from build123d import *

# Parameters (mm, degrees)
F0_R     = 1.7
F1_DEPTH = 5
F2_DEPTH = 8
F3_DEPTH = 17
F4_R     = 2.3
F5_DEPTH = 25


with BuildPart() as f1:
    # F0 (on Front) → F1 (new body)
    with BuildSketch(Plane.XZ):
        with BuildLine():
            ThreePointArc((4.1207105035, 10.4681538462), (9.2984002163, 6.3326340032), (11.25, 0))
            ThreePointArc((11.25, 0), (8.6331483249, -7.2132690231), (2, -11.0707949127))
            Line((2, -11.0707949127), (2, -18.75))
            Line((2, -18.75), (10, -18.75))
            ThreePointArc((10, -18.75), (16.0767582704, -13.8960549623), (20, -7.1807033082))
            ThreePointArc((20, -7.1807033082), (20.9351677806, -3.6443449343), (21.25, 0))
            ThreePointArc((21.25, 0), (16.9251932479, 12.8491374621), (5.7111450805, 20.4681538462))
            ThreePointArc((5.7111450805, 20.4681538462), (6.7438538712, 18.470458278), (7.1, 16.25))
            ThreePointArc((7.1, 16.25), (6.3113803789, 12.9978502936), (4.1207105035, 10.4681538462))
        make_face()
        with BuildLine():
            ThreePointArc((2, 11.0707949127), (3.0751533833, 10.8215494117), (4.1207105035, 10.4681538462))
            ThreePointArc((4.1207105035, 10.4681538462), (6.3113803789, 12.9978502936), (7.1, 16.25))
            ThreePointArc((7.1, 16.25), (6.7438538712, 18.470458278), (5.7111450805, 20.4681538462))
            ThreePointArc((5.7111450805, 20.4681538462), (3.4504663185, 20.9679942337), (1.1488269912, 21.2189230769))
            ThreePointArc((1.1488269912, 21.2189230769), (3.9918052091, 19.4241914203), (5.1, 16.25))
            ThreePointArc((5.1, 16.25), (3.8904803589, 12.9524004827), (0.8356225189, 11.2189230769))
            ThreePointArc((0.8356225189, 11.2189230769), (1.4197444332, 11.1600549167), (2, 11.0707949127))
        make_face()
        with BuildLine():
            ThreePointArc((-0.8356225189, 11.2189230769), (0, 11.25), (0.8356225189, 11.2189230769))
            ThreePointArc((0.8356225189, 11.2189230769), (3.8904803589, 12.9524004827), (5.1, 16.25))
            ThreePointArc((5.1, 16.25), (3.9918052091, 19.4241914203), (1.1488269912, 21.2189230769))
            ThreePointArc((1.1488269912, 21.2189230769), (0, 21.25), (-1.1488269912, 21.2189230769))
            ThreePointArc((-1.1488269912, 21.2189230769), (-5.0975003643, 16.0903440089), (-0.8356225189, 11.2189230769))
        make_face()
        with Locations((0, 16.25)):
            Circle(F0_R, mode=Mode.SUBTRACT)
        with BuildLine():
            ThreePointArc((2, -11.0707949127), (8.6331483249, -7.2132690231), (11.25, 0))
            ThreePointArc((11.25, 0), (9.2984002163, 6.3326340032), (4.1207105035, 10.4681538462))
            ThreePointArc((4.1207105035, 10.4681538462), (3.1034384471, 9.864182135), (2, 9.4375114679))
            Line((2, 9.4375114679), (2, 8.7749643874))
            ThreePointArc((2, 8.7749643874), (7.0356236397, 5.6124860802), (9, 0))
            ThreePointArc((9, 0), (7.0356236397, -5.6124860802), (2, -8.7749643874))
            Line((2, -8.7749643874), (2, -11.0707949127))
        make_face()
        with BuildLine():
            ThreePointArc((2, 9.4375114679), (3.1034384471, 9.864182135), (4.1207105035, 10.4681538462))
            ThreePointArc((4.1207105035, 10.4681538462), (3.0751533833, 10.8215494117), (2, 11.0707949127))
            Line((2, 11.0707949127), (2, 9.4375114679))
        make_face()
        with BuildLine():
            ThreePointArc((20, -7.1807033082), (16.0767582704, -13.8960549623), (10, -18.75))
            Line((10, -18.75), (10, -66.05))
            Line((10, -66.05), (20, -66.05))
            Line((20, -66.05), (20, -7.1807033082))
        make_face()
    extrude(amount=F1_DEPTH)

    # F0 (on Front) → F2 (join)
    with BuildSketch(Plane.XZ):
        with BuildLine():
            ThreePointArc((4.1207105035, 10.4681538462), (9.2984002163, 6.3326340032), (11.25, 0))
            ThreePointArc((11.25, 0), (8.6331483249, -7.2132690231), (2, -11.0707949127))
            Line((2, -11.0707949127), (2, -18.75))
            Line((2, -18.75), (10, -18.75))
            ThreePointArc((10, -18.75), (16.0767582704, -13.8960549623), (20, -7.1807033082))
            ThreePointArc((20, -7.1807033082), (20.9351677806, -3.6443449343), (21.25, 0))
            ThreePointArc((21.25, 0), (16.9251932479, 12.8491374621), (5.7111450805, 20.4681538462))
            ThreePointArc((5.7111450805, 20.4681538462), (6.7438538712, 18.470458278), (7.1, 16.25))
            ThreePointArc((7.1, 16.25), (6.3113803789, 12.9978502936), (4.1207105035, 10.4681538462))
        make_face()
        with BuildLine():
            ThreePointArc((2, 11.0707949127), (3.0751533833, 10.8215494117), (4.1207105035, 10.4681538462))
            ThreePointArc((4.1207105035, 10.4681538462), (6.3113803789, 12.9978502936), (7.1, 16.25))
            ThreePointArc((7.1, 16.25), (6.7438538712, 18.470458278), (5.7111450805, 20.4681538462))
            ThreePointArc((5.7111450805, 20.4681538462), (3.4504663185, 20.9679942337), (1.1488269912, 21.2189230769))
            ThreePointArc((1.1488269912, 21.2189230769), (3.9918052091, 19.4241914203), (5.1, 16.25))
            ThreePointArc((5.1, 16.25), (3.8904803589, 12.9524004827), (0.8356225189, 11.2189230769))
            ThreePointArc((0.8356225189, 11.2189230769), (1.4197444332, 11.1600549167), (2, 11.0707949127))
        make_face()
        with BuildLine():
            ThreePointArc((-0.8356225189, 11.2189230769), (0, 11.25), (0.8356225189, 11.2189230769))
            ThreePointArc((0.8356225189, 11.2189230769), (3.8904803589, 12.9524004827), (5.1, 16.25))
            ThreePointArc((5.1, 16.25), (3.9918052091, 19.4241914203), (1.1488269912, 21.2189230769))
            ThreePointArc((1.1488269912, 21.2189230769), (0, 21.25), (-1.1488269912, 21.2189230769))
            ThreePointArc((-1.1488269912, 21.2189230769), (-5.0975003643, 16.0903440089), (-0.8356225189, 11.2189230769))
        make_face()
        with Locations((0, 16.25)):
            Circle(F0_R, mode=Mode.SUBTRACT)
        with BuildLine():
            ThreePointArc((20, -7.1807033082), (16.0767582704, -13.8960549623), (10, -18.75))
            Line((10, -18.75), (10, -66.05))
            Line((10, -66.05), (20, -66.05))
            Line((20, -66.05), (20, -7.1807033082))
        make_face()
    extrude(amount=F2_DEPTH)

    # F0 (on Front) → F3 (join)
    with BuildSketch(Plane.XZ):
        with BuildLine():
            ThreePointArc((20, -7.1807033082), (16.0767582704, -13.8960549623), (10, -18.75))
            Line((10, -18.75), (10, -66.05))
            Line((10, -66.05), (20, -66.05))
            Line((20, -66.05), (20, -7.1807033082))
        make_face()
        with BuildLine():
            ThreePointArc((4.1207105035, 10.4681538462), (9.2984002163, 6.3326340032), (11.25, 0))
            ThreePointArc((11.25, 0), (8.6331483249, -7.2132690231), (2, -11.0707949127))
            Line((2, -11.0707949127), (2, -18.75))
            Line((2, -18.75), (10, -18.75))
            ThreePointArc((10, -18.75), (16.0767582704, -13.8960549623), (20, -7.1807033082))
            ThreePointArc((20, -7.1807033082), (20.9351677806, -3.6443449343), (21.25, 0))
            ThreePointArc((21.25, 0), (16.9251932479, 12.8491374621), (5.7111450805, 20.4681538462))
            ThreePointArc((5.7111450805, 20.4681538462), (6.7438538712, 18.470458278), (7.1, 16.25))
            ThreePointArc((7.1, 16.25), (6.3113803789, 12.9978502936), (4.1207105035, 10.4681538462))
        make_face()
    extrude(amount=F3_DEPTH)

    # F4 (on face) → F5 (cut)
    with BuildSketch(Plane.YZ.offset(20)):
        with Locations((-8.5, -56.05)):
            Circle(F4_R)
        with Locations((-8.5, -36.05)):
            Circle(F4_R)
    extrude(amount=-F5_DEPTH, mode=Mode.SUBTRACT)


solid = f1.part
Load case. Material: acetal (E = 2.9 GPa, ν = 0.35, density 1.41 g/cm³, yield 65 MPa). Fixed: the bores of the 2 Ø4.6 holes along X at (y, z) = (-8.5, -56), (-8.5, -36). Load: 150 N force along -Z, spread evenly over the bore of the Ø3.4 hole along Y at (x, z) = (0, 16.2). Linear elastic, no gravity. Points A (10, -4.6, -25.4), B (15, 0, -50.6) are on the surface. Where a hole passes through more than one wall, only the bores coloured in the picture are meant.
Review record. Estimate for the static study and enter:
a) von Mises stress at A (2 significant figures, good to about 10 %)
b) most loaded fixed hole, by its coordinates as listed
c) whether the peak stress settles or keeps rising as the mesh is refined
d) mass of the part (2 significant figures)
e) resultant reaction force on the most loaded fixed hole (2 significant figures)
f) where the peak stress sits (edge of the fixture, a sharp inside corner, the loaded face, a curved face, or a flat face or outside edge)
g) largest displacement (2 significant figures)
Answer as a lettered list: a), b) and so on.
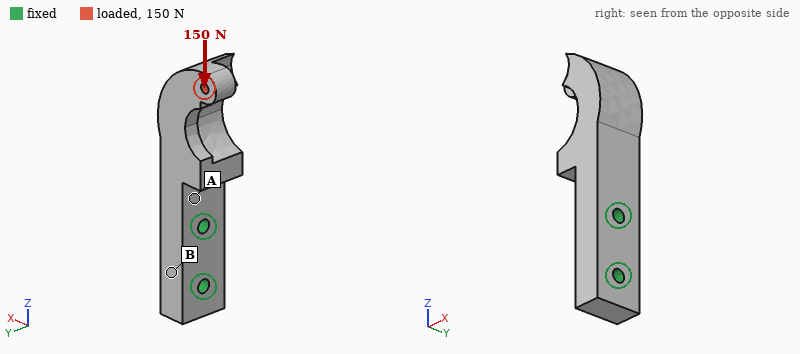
a) 9.5 MPa
b) (-8.5, -36)
c) keeps rising
d) 23 g
e) 140 N
f) edge of the fixture
g) 0.88 mm
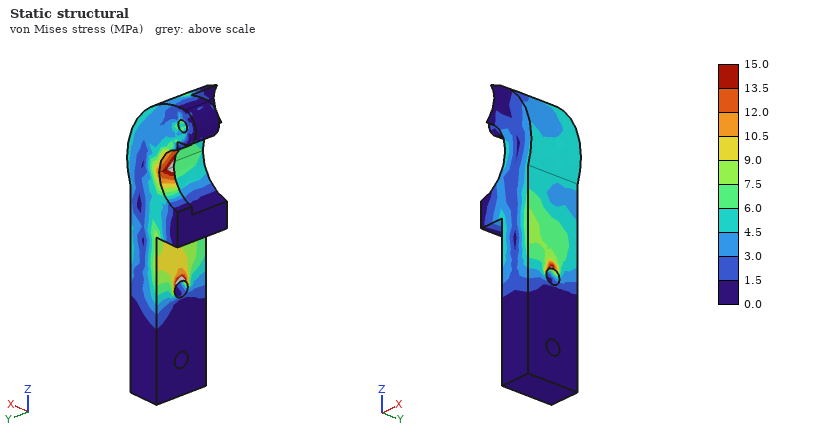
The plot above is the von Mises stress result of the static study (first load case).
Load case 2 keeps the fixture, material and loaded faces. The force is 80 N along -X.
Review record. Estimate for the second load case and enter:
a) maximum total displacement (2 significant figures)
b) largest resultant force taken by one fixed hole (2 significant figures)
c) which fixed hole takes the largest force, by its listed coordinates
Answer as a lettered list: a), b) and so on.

a) 1.1 mm
b) 120 N
c) (-8.5, -36)
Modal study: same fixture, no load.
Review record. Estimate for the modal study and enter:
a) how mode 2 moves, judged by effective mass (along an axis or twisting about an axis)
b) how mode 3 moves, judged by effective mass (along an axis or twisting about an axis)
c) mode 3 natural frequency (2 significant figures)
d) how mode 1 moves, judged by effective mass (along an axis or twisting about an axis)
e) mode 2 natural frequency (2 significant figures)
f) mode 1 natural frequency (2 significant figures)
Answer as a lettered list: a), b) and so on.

a) along Y
b) twisting about Z
c) 2400 Hz
d) along X
e) 890 Hz
f) 660 Hz
